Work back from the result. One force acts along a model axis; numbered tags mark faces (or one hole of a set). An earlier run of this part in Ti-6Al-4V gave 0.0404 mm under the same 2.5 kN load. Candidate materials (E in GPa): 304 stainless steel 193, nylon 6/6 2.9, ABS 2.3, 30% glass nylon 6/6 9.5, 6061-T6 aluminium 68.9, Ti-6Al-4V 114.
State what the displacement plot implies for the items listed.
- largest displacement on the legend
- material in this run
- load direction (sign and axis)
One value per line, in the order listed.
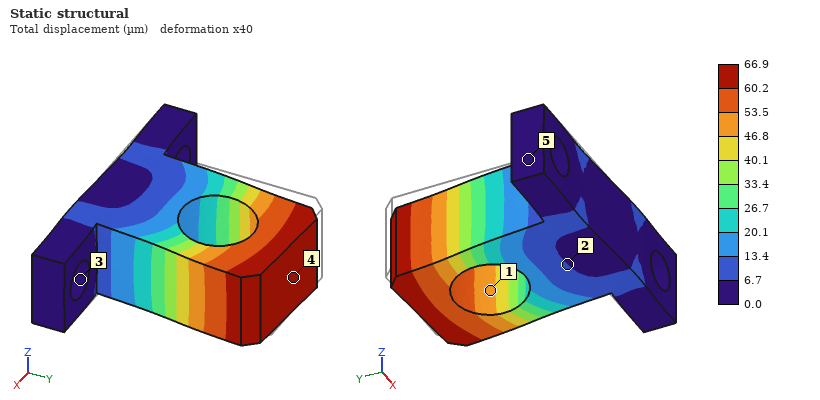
66.9 µm
6061-T6 aluminium
+X
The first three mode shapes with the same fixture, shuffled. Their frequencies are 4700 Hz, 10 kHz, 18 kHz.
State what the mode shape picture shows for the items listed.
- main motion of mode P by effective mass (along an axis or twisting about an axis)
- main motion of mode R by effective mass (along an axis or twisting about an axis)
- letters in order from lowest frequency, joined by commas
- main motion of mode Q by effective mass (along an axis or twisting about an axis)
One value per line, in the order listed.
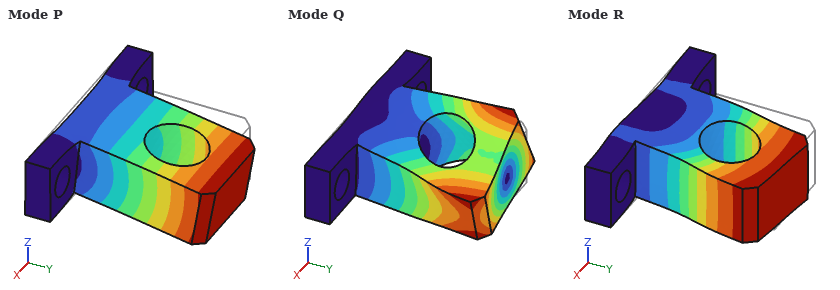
along Z
along X
P, R, Q
twisting about Y
